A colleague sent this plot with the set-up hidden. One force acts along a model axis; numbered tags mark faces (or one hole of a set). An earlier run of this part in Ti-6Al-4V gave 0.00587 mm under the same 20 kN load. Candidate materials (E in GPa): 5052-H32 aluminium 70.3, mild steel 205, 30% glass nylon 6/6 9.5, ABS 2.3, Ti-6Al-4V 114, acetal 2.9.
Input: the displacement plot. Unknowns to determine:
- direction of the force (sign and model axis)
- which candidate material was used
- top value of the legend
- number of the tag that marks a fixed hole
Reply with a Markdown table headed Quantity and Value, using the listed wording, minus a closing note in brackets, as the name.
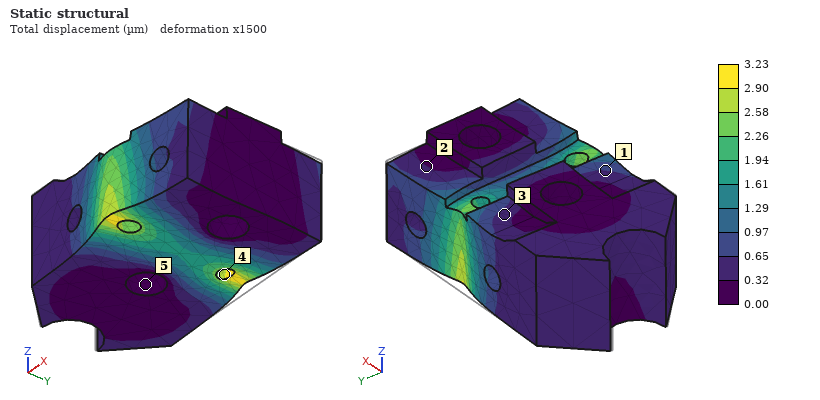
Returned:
| Quantity | Value |
|---|---|
| direction of the force | -Y |
| which candidate material was used | mild steel |
| top value of the legend | 3.23 µm |
| number of the tag that marks a fixed hole | 5 |
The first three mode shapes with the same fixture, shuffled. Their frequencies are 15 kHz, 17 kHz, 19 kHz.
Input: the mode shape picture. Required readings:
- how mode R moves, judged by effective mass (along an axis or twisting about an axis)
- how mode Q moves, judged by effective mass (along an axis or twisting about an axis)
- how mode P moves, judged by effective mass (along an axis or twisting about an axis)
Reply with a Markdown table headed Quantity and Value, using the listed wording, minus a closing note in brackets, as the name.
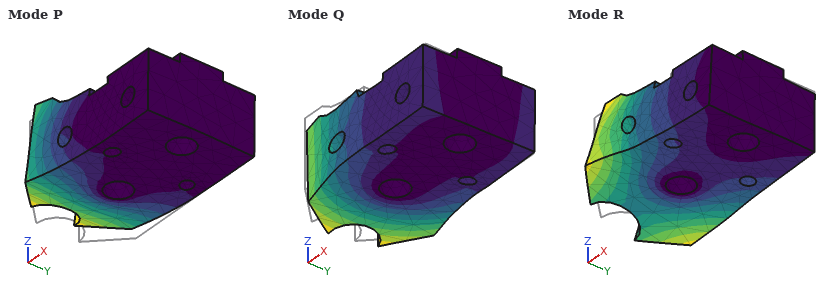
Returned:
| Quantity | Value |
|---|---|
| how mode R moves, judged by effective mass | twisting about X |
| how mode Q moves, judged by effective mass | along Y |
| how mode P moves, judged by effective mass | along Z |
